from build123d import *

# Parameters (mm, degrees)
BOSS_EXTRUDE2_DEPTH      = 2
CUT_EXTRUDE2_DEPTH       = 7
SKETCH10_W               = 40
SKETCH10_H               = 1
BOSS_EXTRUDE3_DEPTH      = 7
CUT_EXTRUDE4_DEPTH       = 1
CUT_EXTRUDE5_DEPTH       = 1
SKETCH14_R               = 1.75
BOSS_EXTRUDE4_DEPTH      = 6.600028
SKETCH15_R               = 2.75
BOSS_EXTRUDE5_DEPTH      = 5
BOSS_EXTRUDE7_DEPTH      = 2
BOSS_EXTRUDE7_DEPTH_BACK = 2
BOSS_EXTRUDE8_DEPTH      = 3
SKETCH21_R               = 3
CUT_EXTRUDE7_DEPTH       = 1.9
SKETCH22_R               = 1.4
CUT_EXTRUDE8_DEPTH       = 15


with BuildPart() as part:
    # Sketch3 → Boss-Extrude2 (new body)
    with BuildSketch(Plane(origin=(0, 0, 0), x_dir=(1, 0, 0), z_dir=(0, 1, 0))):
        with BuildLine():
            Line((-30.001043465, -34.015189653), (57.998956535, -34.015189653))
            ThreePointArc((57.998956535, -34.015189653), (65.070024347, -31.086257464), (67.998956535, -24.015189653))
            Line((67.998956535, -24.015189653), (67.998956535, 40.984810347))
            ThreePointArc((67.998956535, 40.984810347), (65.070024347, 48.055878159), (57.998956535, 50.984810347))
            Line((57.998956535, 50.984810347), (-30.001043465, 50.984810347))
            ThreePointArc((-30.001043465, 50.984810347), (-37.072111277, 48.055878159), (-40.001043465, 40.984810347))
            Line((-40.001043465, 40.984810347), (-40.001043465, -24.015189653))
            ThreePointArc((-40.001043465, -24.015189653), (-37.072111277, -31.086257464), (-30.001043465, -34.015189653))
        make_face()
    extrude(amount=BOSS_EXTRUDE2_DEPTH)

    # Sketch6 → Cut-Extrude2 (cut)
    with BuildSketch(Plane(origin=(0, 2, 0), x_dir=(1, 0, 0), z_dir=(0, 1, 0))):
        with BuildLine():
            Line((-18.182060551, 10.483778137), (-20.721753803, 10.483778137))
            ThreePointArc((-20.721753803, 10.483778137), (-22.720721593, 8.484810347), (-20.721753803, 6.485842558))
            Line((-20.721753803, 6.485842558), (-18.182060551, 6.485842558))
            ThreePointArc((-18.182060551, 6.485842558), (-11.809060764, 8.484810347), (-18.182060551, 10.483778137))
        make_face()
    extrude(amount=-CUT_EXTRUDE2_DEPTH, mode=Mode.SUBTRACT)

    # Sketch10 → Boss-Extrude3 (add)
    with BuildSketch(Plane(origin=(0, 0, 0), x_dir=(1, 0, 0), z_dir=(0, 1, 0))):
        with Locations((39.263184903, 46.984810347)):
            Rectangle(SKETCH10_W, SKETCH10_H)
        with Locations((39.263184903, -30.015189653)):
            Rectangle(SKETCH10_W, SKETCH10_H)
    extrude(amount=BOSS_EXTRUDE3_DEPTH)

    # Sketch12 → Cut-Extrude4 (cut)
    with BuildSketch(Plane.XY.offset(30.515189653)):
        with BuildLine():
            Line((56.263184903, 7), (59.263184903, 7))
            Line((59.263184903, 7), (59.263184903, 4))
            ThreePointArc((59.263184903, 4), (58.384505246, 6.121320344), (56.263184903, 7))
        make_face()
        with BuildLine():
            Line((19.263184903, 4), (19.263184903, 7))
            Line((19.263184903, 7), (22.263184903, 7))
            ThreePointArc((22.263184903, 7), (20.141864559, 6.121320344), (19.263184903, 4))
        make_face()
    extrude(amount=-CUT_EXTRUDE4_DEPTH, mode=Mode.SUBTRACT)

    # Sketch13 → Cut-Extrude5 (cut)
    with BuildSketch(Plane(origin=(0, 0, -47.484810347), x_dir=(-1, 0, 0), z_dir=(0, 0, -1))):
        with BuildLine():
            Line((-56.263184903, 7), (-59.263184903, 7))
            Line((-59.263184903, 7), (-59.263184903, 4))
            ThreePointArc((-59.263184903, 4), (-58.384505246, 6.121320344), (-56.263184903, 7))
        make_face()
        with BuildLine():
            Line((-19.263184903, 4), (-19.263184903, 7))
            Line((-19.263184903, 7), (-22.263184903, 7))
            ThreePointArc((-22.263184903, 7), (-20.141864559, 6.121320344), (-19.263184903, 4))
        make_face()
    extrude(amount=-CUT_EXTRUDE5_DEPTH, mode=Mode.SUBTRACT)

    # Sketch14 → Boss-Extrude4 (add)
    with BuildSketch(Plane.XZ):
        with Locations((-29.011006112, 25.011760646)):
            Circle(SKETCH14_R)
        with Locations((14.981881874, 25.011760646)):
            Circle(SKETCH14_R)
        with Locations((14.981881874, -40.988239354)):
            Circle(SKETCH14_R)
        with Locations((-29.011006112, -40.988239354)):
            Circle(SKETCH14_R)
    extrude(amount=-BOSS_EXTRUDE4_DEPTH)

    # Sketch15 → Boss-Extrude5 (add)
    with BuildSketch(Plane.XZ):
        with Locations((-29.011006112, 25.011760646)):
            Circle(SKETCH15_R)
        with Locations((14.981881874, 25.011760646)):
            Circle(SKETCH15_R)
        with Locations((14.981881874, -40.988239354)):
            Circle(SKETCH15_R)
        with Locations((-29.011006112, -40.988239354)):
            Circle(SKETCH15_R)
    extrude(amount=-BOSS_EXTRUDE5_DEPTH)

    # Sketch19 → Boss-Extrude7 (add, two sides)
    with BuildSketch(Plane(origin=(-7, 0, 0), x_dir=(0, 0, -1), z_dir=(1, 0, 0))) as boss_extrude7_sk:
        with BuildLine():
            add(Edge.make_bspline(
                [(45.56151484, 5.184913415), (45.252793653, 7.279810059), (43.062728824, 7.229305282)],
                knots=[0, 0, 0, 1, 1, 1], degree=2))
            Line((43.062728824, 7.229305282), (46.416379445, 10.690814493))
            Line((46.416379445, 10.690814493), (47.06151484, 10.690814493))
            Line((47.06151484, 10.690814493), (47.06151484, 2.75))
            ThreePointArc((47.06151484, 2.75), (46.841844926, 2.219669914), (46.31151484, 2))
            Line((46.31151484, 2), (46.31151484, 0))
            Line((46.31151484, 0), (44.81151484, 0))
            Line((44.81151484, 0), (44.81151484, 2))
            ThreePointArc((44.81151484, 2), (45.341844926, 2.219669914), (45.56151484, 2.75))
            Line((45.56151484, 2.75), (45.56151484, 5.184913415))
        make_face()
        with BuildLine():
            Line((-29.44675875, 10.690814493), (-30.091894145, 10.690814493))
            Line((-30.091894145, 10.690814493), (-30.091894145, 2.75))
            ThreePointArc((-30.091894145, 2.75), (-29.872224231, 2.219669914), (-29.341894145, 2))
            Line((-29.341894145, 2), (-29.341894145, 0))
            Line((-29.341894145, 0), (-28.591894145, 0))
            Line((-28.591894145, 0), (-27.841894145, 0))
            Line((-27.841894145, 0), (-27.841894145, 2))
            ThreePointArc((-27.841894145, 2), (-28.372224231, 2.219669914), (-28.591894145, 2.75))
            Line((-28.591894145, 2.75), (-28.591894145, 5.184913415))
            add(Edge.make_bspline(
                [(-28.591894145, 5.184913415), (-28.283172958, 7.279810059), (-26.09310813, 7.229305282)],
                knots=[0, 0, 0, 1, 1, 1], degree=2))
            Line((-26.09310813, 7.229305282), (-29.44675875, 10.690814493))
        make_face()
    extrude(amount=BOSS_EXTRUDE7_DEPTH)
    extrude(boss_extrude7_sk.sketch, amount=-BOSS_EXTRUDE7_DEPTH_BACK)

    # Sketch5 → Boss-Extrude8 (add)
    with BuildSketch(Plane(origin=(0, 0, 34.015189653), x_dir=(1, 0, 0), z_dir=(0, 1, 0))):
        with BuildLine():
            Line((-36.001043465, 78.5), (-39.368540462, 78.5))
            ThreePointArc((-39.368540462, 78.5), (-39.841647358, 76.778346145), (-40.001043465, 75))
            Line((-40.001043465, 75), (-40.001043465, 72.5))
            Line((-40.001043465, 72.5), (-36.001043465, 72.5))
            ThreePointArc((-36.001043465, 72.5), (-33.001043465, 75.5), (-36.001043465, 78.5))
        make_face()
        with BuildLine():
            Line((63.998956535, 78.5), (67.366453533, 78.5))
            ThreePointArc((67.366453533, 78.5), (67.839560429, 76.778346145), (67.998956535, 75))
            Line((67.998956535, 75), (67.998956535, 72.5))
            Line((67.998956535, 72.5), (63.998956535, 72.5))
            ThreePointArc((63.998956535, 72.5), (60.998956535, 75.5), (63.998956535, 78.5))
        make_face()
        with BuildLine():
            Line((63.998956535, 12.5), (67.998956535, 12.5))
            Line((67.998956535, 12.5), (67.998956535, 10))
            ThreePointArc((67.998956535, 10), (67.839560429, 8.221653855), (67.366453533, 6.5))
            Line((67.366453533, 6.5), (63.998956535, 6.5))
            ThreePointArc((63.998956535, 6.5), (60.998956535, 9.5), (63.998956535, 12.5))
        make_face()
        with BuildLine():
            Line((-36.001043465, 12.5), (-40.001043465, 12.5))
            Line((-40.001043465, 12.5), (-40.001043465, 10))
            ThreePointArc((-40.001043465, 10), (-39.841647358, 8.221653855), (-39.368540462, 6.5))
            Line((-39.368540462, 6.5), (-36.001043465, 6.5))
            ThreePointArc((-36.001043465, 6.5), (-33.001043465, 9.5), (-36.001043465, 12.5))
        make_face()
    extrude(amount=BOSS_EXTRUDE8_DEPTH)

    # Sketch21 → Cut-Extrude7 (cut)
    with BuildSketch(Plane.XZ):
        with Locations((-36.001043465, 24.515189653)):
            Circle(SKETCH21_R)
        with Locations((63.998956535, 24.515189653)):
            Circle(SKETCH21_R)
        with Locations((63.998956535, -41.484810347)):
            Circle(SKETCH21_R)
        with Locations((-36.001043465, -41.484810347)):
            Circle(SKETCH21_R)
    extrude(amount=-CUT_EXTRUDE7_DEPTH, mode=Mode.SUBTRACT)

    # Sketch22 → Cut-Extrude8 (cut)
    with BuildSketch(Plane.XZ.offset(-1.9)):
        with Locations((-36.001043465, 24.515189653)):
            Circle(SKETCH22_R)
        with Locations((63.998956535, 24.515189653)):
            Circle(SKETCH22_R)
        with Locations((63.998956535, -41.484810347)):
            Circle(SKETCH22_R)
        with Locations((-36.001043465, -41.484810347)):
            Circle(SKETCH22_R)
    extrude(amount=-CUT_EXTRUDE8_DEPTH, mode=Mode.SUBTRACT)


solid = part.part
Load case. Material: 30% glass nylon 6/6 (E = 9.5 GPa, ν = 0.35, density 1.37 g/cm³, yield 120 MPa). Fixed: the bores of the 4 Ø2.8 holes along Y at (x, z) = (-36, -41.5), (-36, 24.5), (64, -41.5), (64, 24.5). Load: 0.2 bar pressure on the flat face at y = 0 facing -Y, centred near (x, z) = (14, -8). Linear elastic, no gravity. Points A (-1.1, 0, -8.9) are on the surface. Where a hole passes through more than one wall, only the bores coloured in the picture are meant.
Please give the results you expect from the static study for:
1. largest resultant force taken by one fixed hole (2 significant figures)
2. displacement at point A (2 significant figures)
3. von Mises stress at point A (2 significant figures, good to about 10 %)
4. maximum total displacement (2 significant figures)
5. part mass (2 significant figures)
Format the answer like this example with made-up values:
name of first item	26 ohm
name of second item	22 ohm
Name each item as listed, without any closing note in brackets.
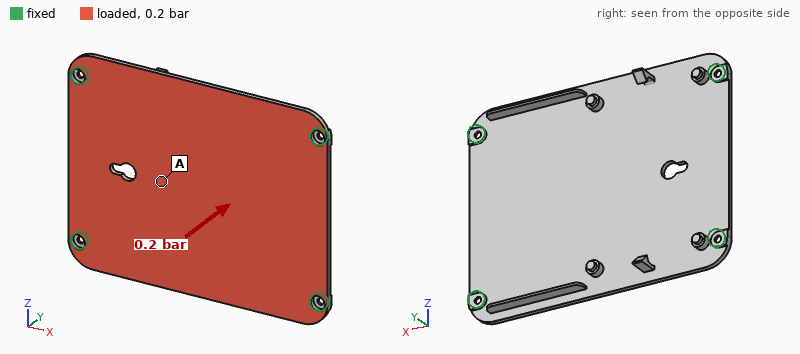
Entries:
largest resultant force taken by one fixed hole	170 N
displacement at point A	1.2 mm
von Mises stress at point A	13 MPa
maximum total displacement	1.4 mm
part mass	26 g
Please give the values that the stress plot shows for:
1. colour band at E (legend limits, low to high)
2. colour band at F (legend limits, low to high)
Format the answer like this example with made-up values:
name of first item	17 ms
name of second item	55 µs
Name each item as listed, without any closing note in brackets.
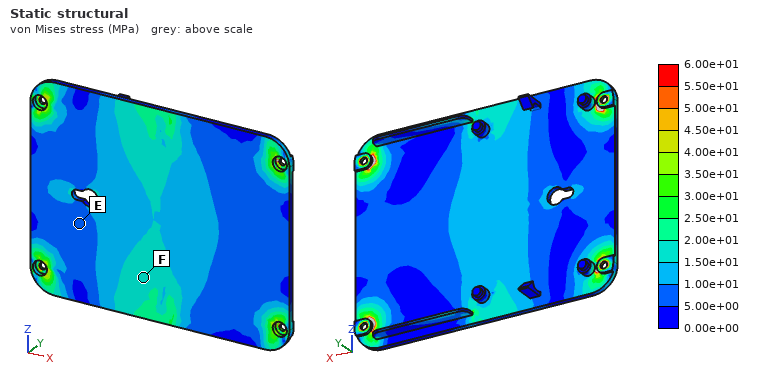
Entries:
colour band at E	5.00e+00 to 1.00e+01 MPa
colour band at F	1.50e+01 to 2.00e+01 MPa
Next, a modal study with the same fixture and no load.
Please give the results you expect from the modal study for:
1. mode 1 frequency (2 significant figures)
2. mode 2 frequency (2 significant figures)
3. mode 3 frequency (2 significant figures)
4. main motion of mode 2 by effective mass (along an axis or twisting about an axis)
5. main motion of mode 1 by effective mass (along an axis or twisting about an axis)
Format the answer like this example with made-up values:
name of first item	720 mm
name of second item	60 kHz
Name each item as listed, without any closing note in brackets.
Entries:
mode 1 frequency	420 Hz
mode 2 frequency	620 Hz
mode 3 frequency	960 Hz
main motion of mode 2 by effective mass	twisting about X
main motion of mode 1 by effective mass	along Y
